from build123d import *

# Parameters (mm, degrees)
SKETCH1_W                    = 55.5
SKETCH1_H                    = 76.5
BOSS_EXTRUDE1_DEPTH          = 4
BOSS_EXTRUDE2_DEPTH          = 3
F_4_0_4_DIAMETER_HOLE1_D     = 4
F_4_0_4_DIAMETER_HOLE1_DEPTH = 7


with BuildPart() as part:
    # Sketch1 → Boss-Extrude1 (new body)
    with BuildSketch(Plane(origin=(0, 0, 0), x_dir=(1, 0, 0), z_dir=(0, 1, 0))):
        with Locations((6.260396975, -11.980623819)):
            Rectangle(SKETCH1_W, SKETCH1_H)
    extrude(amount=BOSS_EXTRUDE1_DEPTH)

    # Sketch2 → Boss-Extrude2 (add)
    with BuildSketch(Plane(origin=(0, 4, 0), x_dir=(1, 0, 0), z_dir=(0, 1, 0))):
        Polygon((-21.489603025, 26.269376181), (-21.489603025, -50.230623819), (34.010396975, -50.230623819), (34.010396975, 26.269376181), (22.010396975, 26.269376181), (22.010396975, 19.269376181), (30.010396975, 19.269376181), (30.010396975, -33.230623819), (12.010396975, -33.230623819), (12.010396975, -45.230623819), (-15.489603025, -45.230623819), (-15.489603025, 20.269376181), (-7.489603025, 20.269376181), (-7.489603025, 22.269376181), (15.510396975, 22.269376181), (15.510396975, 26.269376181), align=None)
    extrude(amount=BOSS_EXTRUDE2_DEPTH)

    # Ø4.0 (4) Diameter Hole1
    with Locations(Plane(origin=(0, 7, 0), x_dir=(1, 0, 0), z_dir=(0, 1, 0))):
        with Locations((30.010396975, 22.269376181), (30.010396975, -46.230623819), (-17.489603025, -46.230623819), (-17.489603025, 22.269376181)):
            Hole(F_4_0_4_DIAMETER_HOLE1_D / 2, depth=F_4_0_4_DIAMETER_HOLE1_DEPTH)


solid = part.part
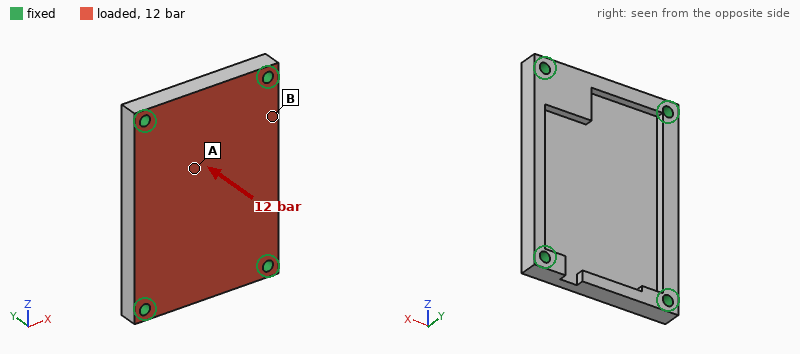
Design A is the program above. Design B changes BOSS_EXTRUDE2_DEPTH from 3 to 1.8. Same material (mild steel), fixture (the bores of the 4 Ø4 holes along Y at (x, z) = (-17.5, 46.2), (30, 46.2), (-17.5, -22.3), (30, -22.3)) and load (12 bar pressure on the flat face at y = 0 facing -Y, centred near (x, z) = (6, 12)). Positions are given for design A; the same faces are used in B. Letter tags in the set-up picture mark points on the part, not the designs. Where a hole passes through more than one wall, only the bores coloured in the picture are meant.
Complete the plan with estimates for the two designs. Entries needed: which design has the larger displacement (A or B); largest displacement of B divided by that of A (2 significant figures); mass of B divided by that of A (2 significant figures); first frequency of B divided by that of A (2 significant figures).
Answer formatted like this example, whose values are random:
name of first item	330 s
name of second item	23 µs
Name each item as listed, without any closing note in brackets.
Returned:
which design has the larger displacement	B
largest displacement of B divided by that of A	1.3
mass of B divided by that of A	0.92
first frequency of B divided by that of A	0.87
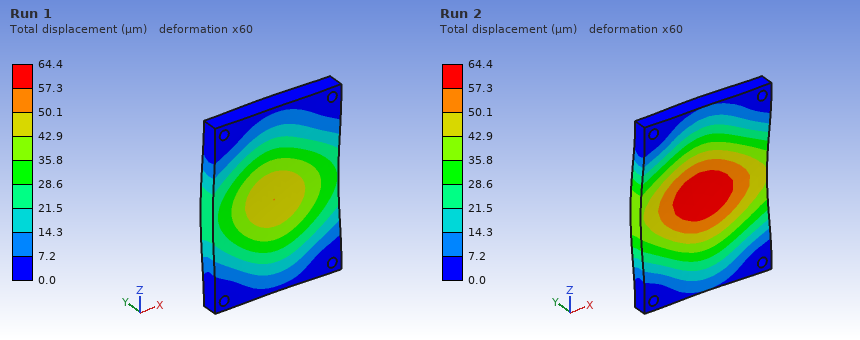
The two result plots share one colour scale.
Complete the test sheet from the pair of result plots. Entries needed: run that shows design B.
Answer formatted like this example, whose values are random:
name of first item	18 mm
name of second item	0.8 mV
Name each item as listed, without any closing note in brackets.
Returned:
run that shows design B	Run 2
